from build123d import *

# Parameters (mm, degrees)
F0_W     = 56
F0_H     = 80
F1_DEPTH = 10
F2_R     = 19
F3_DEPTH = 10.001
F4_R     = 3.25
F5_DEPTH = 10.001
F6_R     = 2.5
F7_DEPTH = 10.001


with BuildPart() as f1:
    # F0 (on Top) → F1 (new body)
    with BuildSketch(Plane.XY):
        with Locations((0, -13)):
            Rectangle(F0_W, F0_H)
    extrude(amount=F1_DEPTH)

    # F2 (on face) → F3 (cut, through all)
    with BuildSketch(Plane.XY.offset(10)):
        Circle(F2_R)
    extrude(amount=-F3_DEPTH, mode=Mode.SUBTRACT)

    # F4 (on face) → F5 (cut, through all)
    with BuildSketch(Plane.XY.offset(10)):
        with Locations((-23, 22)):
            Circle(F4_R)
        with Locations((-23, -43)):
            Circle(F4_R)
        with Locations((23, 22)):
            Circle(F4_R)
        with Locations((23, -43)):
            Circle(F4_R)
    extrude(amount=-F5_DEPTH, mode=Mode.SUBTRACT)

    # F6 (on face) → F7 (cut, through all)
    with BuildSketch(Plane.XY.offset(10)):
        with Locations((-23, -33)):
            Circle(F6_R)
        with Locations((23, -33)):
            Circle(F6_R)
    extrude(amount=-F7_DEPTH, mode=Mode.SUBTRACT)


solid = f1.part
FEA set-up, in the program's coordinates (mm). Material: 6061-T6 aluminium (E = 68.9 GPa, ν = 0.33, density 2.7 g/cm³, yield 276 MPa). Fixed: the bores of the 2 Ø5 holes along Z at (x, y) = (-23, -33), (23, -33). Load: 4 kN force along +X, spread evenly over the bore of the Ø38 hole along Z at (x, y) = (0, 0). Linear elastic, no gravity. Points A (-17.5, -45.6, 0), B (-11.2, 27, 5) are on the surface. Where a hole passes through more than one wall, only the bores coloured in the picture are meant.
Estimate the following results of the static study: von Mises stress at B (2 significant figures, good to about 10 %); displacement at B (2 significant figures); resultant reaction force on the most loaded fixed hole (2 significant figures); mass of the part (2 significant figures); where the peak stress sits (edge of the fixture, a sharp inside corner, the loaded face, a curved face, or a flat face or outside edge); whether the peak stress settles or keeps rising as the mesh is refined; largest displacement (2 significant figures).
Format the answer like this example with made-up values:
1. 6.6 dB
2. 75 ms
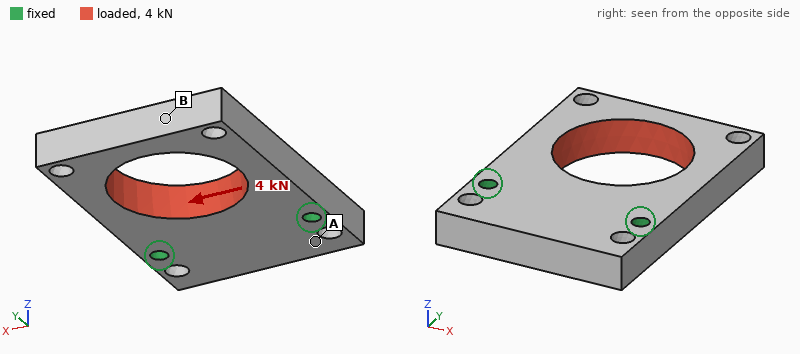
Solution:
1. 30 MPa
2. 0.096 mm
3. 3.4 kN
4. 86 g
5. edge of the fixture
6. keeps rising
7. 0.10 mm
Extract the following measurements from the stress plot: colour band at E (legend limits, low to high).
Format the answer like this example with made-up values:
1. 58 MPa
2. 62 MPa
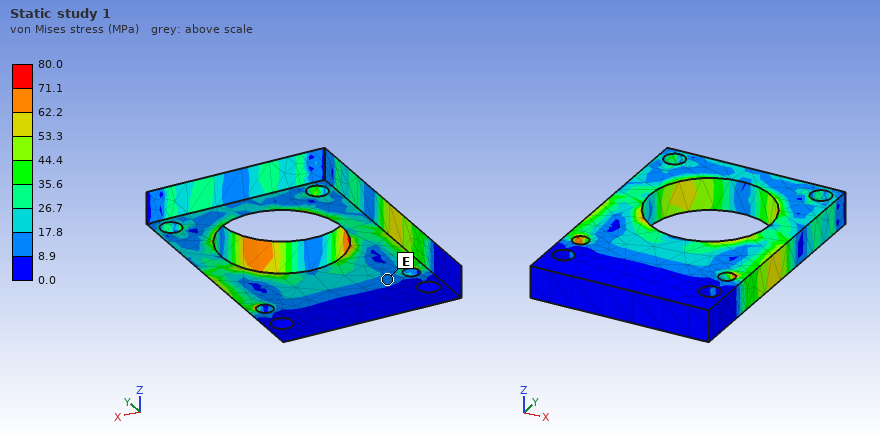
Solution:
1. 8.9 to 17.8 MPa
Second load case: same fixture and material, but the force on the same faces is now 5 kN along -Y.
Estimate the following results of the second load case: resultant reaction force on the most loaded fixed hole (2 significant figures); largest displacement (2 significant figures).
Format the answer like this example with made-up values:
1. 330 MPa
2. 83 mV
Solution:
1. 2.5 kN
2. 26 µm
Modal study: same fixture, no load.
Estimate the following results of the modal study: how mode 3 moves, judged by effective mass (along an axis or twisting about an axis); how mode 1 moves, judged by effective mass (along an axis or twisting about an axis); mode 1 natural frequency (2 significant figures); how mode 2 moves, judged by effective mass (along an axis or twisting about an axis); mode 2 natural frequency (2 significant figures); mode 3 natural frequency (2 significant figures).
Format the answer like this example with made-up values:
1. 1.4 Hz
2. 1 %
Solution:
1. along X
2. along Z
3. 2000 Hz
4. twisting about Y
5. 4400 Hz
6. 5100 Hz
